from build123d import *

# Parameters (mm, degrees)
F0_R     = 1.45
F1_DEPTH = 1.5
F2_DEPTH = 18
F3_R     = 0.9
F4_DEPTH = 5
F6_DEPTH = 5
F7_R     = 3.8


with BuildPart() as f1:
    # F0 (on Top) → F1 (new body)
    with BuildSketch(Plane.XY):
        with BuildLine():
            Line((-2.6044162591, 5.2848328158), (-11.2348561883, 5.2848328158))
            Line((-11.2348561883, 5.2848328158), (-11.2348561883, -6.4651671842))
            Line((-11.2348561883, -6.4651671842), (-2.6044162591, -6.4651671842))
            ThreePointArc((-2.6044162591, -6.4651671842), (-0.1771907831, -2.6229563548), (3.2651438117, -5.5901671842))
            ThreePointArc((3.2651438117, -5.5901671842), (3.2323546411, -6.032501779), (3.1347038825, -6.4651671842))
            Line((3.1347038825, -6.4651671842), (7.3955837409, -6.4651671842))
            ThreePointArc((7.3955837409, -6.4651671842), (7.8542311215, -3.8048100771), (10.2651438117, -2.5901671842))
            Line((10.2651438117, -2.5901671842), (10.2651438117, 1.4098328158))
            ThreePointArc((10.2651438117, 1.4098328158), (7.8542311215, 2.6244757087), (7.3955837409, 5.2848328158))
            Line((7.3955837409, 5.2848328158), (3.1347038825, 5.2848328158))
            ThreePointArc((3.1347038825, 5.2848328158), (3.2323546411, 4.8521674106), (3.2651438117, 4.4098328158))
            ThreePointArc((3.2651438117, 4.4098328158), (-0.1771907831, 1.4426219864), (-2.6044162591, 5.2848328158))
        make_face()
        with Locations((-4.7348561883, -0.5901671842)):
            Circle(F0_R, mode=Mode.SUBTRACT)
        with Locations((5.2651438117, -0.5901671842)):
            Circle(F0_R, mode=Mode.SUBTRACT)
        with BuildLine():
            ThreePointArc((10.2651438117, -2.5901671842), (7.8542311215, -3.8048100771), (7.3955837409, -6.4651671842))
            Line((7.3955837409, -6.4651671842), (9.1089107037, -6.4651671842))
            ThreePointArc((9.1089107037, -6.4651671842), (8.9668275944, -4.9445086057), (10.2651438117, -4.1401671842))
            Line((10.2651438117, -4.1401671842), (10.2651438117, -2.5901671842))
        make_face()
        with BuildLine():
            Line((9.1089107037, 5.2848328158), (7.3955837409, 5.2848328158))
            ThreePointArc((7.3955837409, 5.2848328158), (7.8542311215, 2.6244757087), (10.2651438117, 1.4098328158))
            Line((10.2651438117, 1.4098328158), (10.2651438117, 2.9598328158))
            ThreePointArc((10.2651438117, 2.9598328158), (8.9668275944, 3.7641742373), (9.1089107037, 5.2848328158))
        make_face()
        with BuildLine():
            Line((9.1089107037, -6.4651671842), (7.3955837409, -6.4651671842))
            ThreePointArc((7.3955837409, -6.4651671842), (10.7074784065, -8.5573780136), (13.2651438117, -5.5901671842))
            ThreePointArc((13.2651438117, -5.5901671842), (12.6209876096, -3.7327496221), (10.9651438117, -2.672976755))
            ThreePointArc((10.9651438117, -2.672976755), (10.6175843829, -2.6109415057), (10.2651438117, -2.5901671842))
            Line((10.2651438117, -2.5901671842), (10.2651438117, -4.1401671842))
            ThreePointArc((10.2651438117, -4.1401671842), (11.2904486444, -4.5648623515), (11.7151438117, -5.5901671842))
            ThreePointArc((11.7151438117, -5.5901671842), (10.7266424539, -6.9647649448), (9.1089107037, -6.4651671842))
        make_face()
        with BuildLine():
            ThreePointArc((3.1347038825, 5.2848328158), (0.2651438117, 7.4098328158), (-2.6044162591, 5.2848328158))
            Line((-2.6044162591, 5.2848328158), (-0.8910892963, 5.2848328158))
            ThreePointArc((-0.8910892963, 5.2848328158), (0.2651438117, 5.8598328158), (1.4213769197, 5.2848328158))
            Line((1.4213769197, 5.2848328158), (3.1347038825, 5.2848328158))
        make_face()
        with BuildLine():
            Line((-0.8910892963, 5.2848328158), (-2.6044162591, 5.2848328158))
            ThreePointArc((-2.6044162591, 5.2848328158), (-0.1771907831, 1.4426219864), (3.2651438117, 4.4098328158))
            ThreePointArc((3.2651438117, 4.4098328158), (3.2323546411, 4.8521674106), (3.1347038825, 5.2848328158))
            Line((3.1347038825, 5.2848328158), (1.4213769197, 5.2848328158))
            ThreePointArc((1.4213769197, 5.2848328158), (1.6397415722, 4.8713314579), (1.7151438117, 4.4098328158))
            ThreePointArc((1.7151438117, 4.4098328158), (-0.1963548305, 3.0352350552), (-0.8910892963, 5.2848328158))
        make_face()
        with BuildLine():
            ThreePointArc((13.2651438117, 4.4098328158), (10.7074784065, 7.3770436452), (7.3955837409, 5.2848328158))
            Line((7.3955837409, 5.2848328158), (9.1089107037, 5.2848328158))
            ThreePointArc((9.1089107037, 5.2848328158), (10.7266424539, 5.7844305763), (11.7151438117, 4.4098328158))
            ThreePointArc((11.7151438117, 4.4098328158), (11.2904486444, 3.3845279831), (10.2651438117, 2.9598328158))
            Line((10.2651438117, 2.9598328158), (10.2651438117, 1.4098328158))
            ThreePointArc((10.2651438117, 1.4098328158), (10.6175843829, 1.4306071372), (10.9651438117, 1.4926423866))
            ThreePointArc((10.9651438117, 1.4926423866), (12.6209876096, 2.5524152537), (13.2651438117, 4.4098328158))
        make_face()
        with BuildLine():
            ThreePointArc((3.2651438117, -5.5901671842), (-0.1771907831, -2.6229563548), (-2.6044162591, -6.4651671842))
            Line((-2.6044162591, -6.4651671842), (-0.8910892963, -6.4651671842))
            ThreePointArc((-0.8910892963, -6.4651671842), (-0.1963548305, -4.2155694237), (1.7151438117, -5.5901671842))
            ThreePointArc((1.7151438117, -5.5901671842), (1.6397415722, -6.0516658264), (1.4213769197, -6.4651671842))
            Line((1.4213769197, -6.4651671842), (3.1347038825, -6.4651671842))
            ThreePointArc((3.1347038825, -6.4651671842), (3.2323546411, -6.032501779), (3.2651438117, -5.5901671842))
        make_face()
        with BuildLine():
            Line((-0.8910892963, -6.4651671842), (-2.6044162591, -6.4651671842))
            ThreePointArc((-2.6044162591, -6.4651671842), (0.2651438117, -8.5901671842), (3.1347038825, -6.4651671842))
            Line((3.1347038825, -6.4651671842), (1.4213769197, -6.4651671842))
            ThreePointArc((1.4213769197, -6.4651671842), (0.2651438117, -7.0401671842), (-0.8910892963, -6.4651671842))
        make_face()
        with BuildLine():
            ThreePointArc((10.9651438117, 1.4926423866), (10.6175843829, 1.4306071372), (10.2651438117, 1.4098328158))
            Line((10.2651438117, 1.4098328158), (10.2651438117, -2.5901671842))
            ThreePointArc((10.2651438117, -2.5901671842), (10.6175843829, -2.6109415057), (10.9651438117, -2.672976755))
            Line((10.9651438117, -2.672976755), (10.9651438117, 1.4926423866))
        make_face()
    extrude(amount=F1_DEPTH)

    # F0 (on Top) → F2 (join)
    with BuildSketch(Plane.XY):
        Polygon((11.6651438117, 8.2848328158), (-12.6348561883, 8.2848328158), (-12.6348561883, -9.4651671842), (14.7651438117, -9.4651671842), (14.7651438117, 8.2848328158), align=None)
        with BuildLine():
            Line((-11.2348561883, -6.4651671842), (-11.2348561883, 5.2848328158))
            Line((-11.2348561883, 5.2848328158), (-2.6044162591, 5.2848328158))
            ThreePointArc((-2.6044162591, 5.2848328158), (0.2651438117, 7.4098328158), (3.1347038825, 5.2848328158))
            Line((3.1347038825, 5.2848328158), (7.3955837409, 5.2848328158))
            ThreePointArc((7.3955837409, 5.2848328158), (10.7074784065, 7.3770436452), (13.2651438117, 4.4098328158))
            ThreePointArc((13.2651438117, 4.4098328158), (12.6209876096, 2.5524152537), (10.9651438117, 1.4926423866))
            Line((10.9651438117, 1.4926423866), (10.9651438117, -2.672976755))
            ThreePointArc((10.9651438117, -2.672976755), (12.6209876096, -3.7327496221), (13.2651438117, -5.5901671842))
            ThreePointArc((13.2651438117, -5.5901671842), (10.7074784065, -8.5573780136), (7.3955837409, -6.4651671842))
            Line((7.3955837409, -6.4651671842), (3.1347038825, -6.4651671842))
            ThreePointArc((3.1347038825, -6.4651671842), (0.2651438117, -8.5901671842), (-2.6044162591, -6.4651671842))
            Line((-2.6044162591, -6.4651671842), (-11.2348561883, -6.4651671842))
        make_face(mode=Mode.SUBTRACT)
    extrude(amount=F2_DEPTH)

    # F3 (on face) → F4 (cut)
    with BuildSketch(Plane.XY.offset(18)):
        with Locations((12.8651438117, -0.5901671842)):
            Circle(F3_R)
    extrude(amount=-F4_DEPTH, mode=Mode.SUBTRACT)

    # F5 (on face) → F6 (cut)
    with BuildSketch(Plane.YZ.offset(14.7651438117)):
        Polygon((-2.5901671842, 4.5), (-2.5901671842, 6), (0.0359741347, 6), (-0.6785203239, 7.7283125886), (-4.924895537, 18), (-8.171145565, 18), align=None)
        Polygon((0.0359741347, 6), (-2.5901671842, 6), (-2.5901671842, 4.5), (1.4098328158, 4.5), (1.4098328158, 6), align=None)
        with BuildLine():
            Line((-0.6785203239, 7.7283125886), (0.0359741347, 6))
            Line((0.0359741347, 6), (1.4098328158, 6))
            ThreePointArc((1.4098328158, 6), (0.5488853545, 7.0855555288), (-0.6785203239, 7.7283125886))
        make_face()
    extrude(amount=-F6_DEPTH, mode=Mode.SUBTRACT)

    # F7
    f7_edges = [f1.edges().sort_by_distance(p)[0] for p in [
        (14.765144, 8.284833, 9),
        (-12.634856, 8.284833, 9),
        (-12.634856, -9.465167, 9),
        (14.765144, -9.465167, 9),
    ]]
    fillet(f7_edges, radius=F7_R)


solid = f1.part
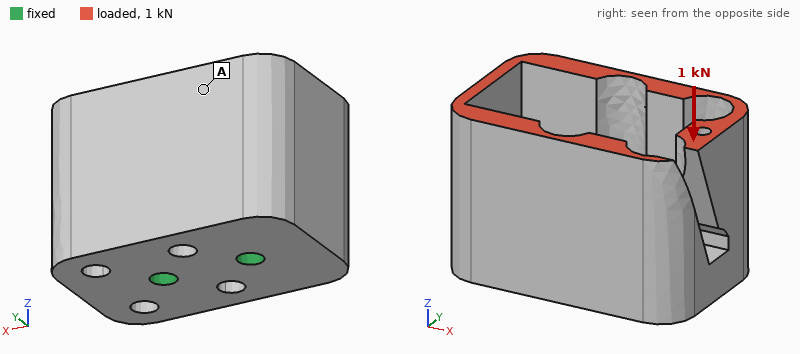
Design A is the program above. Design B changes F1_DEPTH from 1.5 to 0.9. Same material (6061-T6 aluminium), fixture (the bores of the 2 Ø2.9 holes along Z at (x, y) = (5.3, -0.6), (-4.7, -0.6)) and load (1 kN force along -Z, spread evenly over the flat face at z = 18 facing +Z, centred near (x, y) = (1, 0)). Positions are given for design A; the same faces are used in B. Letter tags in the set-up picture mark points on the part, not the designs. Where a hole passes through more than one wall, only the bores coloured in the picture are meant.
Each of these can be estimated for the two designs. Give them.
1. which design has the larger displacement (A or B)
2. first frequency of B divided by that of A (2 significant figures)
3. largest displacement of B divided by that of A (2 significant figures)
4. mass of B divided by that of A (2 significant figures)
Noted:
B
0.56
2.5
0.95
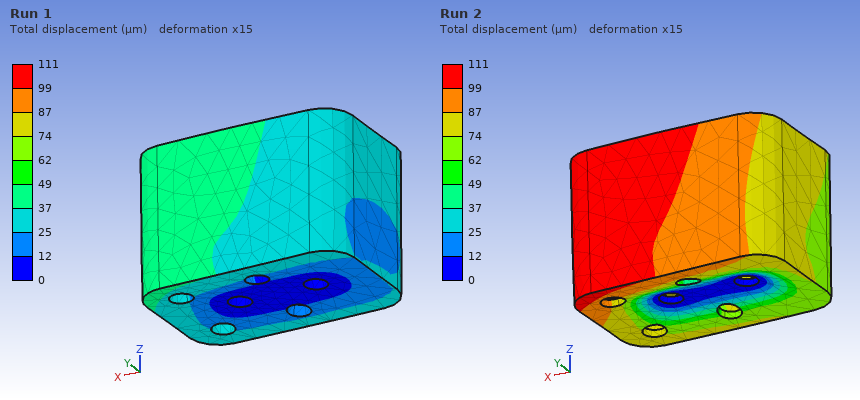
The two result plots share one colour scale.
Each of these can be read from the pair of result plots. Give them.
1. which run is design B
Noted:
Run 2
